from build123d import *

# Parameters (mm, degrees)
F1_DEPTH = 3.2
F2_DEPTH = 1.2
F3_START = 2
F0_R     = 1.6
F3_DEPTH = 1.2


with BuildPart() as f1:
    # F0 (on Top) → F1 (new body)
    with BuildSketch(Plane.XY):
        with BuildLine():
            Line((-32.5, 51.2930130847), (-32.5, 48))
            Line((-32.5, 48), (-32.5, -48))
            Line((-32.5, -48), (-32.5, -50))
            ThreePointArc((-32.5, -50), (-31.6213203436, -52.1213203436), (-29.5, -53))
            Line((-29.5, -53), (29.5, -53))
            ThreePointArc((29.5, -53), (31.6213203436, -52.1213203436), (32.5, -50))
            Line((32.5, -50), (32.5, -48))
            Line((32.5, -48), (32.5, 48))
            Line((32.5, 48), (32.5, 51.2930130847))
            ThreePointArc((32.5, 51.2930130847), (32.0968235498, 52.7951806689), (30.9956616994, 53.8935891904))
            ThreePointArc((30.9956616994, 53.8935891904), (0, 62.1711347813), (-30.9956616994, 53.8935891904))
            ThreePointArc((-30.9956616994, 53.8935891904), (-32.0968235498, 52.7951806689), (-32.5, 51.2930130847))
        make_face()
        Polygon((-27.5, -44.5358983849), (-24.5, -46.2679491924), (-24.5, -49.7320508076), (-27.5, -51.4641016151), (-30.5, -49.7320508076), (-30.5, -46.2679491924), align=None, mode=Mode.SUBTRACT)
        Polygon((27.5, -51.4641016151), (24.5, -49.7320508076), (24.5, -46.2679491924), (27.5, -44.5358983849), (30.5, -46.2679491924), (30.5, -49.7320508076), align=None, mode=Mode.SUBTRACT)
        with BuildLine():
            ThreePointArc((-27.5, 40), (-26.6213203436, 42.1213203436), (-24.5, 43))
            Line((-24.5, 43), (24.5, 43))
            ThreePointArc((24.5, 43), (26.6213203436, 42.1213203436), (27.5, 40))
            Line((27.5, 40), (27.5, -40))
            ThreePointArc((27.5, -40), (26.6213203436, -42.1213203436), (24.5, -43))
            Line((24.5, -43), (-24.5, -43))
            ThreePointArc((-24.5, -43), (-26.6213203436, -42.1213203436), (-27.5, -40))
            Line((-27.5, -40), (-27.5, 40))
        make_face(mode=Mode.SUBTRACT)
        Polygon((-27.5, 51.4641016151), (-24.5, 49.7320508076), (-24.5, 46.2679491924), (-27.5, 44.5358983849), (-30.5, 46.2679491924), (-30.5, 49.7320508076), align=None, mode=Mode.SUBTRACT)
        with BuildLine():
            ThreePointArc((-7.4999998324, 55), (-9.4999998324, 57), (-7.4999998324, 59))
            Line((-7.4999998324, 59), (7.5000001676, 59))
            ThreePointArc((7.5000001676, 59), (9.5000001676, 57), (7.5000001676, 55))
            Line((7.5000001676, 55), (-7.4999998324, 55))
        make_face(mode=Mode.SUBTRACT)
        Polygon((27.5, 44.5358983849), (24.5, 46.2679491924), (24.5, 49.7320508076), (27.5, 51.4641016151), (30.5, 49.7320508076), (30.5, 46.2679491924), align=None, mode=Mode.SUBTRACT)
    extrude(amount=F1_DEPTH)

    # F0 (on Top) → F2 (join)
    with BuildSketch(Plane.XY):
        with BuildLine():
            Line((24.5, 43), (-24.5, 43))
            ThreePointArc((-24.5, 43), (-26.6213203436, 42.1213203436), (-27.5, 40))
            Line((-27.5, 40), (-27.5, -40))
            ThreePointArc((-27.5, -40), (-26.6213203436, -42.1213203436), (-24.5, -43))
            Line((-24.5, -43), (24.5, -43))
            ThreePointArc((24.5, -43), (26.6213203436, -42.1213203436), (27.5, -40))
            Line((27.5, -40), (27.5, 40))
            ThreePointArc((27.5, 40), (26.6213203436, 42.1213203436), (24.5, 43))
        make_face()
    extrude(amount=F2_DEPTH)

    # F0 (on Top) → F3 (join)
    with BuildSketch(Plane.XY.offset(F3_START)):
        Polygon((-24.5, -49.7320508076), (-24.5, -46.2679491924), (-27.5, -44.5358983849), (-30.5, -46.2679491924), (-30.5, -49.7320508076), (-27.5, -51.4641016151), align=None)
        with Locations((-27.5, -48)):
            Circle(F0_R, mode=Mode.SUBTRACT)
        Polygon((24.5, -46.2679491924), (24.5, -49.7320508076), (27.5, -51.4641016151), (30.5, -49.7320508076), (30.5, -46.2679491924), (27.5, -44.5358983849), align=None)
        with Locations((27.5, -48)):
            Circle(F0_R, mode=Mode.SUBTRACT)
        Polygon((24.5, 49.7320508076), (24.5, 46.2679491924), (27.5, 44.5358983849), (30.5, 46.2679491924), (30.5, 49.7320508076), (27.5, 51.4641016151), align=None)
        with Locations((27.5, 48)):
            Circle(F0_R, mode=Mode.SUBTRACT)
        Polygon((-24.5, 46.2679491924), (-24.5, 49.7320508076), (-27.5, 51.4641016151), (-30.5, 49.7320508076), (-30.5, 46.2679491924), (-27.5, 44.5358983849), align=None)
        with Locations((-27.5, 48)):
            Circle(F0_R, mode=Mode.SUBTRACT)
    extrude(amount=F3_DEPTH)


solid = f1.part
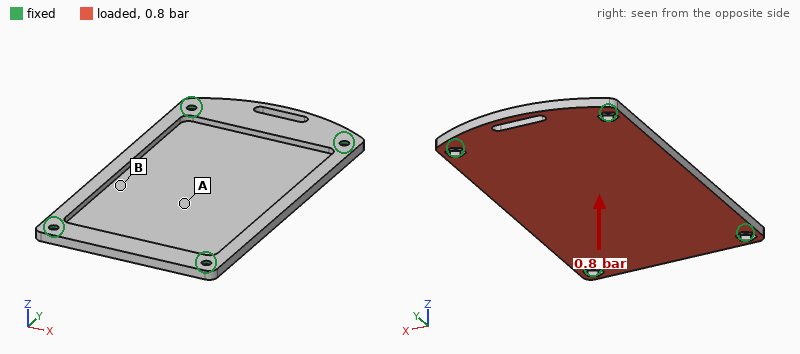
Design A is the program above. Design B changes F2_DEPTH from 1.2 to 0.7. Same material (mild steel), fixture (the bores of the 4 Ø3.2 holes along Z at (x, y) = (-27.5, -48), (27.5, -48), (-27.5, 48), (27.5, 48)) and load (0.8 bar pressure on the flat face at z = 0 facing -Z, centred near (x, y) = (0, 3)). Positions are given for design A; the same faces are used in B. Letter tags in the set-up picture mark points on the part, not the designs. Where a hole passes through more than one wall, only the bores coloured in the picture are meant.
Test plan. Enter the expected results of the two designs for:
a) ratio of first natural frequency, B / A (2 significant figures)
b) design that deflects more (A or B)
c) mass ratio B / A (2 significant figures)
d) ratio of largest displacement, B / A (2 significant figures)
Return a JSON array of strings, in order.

["0.92", "B", "0.82", "2.3"]
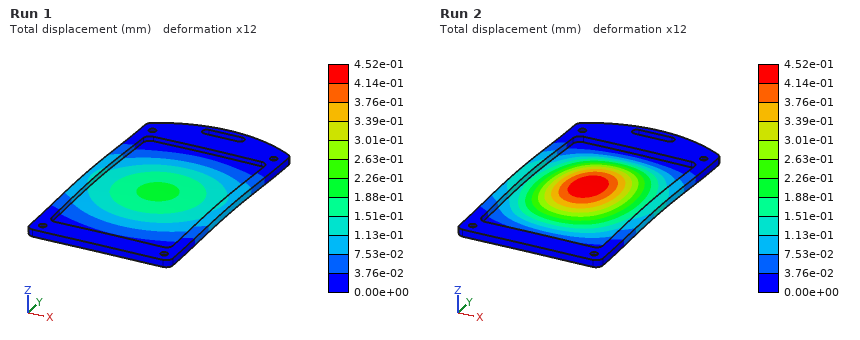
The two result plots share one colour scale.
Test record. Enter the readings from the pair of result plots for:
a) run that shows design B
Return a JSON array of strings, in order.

["Run 2"]
